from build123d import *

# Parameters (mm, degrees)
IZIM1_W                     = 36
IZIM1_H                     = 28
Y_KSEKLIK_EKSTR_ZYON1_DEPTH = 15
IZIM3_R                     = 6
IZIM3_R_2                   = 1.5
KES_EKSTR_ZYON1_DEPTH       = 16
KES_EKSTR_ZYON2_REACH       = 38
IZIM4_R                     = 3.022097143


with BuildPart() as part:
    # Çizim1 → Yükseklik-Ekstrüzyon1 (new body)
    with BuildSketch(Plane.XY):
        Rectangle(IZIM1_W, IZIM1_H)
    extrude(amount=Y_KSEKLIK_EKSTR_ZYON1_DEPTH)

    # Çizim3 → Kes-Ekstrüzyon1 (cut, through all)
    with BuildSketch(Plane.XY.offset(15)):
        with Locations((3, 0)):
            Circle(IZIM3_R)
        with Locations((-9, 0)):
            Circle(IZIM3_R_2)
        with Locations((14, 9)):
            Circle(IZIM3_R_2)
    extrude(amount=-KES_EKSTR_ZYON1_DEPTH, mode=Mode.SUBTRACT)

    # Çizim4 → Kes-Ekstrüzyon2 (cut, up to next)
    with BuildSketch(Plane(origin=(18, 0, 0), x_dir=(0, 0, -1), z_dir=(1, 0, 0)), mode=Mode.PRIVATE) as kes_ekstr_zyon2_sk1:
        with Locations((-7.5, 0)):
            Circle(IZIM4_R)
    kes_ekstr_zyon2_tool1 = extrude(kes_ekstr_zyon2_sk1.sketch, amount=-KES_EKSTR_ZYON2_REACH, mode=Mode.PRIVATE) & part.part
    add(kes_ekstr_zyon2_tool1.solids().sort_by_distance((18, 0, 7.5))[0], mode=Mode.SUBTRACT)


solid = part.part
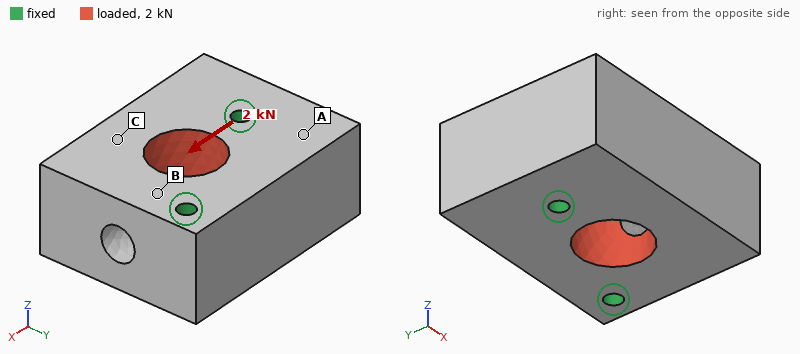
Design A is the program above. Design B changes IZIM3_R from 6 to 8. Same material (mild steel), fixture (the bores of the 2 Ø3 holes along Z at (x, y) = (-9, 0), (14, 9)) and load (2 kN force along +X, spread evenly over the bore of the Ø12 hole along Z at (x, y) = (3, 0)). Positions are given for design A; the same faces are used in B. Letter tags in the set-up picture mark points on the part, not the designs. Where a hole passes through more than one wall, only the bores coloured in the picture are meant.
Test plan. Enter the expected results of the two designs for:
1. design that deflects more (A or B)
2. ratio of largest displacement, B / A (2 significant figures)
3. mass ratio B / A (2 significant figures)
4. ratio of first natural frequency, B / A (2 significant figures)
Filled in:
B
1.5
0.90
0.95
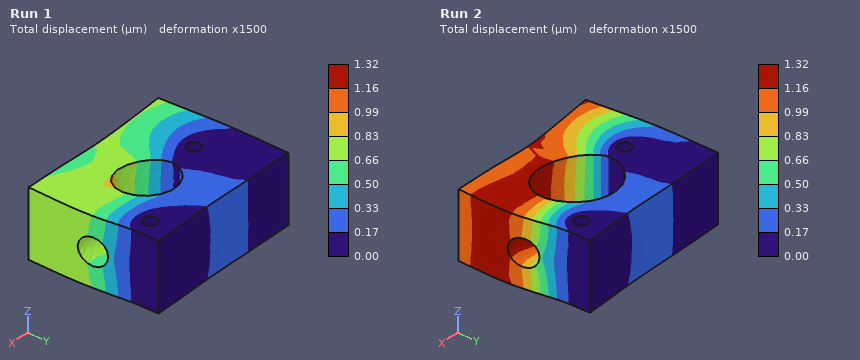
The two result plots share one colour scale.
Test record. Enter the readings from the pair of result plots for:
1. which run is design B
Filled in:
Run 2
